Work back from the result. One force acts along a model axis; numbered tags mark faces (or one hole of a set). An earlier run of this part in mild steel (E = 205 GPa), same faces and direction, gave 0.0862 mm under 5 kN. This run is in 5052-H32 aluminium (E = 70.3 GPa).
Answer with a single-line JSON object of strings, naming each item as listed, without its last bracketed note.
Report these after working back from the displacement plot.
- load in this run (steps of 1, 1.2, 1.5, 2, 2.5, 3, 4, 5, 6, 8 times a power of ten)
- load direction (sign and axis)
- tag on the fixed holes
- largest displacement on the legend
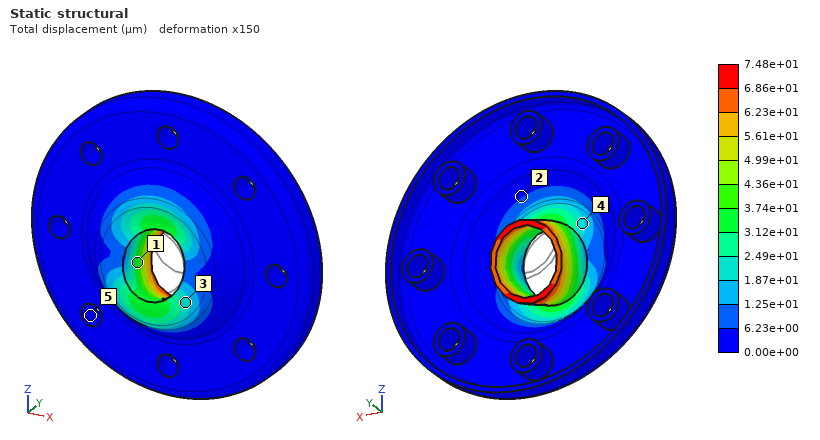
{"load in this run": "1.5 kN", "load direction": "-Z", "tag on the fixed holes": "5", "largest displacement on the legend": "7.48e+01 µm"}
